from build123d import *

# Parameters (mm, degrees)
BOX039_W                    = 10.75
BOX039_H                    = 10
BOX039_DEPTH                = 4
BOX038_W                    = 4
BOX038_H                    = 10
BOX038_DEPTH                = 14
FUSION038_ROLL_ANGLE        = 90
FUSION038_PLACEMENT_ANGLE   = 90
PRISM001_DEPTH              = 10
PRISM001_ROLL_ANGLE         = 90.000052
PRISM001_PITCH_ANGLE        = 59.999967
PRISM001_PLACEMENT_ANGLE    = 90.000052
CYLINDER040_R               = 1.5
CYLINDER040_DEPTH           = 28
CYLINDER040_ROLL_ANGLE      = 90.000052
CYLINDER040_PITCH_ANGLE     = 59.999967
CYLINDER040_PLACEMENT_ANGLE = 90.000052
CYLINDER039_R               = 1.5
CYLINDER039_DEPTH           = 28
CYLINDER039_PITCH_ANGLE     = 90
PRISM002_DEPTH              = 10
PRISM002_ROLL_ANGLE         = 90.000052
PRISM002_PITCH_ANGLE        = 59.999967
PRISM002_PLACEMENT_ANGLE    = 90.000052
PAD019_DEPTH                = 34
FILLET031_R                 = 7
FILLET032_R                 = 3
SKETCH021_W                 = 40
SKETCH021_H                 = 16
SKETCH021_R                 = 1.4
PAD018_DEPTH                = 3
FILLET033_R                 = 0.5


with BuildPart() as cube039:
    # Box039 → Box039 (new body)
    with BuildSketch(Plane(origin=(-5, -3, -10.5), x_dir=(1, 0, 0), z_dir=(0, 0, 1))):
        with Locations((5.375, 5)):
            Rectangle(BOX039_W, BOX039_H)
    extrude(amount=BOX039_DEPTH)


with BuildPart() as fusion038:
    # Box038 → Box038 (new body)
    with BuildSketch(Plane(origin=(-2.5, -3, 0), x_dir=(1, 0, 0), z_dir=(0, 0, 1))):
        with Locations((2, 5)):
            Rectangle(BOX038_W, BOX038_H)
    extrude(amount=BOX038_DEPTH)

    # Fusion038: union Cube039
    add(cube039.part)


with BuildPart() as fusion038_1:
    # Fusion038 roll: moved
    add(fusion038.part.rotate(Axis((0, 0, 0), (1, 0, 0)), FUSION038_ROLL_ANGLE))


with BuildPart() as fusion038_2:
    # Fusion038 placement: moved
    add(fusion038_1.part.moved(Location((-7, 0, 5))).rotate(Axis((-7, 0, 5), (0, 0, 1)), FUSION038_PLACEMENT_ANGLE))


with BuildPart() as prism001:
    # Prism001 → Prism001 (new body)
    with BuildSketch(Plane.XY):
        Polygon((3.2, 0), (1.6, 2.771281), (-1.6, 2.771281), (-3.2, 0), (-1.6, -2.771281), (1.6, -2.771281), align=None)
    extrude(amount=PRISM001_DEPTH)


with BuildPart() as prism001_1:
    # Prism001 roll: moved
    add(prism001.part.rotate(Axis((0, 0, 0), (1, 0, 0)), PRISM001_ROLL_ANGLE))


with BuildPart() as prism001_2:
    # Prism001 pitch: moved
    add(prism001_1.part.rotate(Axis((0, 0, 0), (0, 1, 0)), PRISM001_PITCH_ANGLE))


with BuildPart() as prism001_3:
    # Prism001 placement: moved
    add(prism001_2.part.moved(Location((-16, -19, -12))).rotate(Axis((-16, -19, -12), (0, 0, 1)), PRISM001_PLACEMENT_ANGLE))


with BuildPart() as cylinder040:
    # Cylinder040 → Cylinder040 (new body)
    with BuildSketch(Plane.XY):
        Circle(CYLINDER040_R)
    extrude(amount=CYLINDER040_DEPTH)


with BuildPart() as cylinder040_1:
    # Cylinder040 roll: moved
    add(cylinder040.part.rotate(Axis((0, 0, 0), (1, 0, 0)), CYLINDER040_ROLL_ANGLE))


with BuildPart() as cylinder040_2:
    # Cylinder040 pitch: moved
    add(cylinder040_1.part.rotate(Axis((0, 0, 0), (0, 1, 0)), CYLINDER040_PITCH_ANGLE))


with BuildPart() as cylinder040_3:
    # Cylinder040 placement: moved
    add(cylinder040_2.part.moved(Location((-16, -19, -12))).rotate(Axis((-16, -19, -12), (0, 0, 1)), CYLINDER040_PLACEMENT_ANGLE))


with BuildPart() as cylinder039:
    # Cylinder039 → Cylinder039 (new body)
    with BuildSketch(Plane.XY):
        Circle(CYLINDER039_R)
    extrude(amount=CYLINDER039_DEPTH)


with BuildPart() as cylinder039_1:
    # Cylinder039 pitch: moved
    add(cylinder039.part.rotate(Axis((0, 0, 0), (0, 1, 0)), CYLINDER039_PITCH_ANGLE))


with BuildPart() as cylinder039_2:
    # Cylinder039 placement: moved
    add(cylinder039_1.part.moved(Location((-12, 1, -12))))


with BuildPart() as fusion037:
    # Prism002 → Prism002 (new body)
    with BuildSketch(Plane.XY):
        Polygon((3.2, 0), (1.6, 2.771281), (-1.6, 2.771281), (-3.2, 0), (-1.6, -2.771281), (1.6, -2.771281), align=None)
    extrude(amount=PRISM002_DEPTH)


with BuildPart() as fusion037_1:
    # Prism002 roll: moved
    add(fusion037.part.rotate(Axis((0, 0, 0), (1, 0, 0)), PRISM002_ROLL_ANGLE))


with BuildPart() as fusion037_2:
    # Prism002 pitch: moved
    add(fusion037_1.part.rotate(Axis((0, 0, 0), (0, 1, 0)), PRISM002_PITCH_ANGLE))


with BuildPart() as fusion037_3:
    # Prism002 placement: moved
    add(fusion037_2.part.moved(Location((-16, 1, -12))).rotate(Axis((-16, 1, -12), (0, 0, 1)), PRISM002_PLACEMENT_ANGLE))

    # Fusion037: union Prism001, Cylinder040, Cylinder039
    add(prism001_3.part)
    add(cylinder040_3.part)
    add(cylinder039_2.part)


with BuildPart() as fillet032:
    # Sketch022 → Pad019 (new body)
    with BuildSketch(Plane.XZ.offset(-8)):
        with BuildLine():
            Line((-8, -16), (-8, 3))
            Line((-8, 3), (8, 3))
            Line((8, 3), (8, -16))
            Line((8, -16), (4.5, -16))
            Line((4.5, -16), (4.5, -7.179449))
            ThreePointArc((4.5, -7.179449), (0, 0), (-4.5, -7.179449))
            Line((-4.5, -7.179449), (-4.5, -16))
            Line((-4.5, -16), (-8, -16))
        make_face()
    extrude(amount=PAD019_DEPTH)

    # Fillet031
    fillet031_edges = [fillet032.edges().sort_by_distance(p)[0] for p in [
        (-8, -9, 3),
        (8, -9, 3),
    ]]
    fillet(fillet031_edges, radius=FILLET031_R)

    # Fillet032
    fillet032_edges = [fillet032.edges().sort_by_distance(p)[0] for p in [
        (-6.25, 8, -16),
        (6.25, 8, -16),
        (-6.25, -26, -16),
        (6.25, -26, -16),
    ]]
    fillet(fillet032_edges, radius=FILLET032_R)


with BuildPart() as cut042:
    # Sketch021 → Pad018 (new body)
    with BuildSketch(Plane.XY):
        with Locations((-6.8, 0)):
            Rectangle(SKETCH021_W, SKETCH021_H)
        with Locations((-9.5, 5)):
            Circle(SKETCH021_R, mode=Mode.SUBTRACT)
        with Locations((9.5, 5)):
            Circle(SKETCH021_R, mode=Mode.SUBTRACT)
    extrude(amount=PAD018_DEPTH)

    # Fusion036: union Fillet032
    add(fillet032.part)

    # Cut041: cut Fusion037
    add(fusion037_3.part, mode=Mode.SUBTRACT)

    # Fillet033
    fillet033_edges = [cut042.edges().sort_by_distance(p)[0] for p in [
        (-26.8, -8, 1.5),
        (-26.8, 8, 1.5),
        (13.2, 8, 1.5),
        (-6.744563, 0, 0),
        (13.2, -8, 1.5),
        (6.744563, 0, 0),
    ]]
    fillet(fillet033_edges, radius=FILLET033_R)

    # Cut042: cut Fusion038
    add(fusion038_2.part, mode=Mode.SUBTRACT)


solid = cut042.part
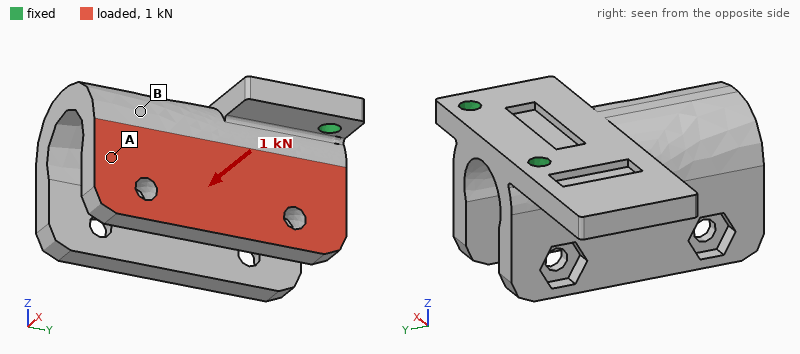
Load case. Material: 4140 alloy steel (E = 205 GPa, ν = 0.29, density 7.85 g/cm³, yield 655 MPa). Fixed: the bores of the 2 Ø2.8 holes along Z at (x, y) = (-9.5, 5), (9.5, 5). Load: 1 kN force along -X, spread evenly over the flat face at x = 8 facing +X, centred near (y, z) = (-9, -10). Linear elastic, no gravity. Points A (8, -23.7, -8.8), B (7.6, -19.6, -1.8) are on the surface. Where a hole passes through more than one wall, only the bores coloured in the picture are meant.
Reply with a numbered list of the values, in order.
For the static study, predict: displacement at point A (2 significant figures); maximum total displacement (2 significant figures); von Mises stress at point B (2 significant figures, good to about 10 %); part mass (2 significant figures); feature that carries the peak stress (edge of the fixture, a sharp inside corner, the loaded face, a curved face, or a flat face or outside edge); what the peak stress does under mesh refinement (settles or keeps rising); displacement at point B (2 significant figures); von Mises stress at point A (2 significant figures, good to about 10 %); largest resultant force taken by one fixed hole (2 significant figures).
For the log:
1. 0.066 mm
2. 0.11 mm
3. 69 MPa
4. 47 g
5. a sharp inside corner
6. keeps rising
7. 0.028 mm
8. 24 MPa
9. 1.1 kN
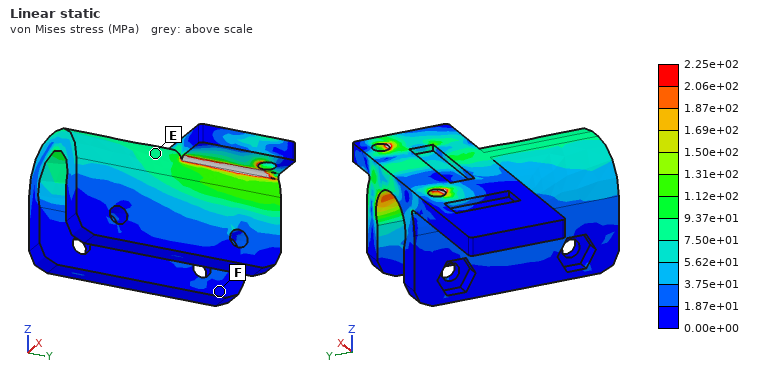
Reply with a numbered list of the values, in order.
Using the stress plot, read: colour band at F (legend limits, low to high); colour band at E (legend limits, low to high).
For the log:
1. 0.00e+00 to 1.87e+01 MPa
2. 7.50e+01 to 9.37e+01 MPa
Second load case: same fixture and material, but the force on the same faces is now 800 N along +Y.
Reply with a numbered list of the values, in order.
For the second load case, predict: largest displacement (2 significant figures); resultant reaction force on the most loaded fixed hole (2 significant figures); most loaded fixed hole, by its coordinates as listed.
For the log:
1. 83 µm
2. 740 N
3. (9.5, 5)
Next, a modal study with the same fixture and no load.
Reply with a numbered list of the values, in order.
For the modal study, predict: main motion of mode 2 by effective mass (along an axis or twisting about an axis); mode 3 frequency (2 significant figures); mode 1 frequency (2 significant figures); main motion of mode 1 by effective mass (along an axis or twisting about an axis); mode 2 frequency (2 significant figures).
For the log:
1. along X
2. 6400 Hz
3. 2800 Hz
4. along Z
5. 4900 Hz
